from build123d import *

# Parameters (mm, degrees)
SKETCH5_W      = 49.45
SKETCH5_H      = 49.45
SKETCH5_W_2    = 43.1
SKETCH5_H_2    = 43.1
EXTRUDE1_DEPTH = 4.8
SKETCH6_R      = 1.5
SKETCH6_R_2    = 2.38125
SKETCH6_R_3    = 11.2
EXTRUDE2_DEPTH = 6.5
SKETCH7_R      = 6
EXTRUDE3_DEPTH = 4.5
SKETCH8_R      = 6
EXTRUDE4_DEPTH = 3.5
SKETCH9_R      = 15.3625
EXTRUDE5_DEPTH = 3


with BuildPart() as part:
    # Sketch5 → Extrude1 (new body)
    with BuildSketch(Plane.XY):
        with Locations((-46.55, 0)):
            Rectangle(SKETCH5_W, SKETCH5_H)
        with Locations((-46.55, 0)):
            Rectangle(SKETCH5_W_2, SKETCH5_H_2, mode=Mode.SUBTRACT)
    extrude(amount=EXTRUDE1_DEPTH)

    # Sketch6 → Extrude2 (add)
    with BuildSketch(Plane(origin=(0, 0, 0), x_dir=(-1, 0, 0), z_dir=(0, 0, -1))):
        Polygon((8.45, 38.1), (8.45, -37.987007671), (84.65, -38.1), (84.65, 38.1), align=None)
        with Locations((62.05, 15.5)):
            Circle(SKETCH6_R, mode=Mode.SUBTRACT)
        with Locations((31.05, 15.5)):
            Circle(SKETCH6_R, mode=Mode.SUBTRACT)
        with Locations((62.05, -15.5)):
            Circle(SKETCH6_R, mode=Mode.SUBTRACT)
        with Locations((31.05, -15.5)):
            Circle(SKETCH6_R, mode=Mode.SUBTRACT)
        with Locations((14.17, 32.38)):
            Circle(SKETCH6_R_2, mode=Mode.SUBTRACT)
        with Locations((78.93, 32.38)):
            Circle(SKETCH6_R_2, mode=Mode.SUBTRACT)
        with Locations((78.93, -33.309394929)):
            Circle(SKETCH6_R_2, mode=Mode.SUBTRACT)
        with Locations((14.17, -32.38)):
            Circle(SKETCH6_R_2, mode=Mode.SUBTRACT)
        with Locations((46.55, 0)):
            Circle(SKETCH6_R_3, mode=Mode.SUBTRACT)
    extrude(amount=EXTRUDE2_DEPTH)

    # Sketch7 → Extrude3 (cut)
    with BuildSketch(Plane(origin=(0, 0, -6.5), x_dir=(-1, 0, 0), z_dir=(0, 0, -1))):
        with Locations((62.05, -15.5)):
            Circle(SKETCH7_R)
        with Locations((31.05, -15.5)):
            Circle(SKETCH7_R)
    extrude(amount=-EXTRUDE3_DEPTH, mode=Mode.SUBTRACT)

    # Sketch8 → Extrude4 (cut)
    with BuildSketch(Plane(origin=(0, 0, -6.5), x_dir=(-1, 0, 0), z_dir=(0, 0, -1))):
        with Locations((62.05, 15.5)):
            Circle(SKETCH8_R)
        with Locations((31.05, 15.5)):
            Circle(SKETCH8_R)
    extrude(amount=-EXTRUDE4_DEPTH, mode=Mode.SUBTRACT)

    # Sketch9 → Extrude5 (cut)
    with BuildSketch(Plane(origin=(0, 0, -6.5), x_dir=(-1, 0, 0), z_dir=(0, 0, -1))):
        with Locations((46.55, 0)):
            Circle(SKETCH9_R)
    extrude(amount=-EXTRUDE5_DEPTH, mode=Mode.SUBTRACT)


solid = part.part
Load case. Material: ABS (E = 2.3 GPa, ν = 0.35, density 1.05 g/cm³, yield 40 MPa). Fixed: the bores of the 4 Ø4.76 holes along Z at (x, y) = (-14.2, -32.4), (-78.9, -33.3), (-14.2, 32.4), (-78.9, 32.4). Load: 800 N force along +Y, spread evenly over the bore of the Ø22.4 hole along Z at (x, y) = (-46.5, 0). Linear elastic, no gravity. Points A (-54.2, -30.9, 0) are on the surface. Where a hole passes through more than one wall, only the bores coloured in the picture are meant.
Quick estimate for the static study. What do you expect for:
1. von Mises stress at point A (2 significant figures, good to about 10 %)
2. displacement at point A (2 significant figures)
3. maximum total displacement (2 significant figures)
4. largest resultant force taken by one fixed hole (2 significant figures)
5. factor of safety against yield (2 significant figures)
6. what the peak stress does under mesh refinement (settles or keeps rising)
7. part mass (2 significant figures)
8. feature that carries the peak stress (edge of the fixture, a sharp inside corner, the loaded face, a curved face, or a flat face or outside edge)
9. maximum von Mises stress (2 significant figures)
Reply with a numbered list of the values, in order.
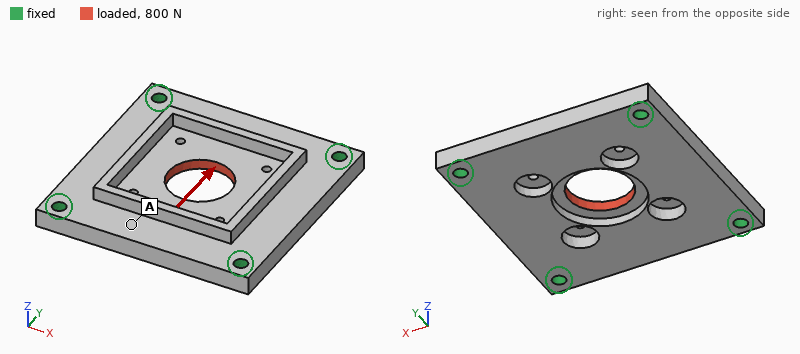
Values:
1. 0.98 MPa
2. 38 µm
3. 57 µm
4. 230 N
5. 4.6
6. settles
7. 36 g
8. a curved face
9. 8.6 MPa
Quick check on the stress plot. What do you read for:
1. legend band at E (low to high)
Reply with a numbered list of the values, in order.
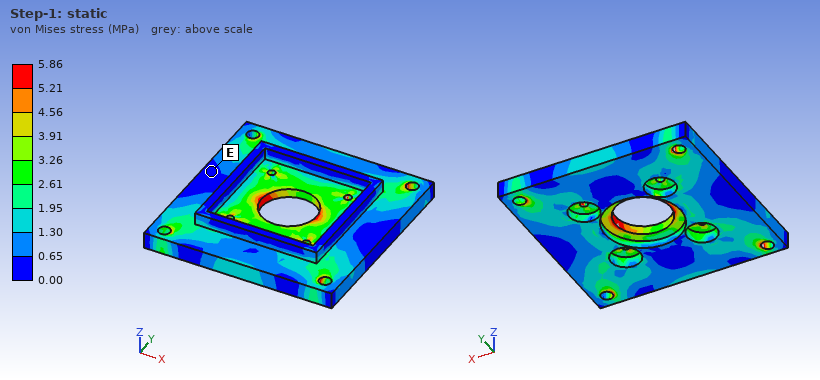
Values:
1. 0.00 to 0.65 MPa
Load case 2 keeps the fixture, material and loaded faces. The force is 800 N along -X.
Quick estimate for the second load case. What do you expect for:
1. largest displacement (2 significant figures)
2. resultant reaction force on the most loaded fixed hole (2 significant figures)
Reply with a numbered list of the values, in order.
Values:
1. 57 µm
2. 230 N
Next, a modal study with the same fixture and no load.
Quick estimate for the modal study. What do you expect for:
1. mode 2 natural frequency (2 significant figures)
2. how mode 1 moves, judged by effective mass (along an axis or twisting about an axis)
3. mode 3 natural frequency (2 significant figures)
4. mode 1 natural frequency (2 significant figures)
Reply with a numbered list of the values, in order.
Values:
1. 2400 Hz
2. along Z
3. 2500 Hz
4. 1600 Hz
